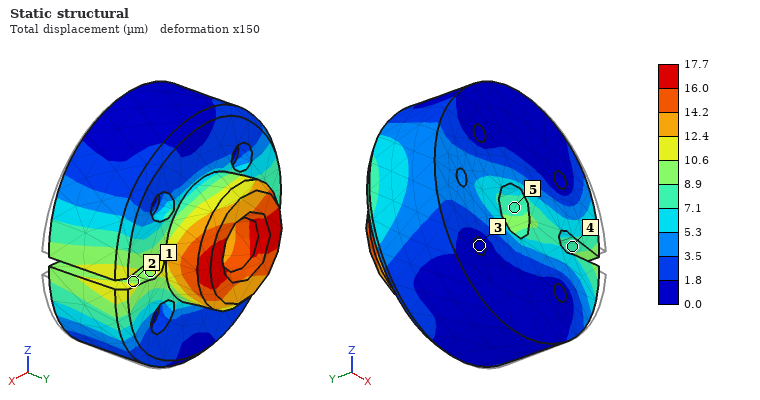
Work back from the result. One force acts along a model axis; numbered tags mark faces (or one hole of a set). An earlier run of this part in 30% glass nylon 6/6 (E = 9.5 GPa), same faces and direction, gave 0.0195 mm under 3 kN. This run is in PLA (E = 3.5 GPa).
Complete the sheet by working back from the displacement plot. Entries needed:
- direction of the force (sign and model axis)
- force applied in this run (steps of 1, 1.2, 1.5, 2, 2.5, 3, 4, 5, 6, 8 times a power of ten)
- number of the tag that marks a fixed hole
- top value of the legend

-X
1 kN
3
17.7 µm
